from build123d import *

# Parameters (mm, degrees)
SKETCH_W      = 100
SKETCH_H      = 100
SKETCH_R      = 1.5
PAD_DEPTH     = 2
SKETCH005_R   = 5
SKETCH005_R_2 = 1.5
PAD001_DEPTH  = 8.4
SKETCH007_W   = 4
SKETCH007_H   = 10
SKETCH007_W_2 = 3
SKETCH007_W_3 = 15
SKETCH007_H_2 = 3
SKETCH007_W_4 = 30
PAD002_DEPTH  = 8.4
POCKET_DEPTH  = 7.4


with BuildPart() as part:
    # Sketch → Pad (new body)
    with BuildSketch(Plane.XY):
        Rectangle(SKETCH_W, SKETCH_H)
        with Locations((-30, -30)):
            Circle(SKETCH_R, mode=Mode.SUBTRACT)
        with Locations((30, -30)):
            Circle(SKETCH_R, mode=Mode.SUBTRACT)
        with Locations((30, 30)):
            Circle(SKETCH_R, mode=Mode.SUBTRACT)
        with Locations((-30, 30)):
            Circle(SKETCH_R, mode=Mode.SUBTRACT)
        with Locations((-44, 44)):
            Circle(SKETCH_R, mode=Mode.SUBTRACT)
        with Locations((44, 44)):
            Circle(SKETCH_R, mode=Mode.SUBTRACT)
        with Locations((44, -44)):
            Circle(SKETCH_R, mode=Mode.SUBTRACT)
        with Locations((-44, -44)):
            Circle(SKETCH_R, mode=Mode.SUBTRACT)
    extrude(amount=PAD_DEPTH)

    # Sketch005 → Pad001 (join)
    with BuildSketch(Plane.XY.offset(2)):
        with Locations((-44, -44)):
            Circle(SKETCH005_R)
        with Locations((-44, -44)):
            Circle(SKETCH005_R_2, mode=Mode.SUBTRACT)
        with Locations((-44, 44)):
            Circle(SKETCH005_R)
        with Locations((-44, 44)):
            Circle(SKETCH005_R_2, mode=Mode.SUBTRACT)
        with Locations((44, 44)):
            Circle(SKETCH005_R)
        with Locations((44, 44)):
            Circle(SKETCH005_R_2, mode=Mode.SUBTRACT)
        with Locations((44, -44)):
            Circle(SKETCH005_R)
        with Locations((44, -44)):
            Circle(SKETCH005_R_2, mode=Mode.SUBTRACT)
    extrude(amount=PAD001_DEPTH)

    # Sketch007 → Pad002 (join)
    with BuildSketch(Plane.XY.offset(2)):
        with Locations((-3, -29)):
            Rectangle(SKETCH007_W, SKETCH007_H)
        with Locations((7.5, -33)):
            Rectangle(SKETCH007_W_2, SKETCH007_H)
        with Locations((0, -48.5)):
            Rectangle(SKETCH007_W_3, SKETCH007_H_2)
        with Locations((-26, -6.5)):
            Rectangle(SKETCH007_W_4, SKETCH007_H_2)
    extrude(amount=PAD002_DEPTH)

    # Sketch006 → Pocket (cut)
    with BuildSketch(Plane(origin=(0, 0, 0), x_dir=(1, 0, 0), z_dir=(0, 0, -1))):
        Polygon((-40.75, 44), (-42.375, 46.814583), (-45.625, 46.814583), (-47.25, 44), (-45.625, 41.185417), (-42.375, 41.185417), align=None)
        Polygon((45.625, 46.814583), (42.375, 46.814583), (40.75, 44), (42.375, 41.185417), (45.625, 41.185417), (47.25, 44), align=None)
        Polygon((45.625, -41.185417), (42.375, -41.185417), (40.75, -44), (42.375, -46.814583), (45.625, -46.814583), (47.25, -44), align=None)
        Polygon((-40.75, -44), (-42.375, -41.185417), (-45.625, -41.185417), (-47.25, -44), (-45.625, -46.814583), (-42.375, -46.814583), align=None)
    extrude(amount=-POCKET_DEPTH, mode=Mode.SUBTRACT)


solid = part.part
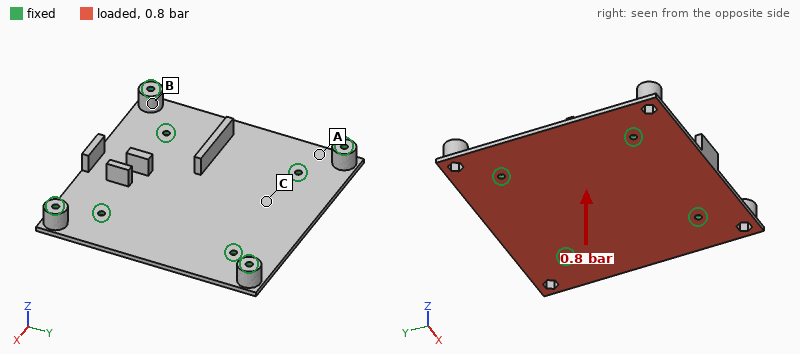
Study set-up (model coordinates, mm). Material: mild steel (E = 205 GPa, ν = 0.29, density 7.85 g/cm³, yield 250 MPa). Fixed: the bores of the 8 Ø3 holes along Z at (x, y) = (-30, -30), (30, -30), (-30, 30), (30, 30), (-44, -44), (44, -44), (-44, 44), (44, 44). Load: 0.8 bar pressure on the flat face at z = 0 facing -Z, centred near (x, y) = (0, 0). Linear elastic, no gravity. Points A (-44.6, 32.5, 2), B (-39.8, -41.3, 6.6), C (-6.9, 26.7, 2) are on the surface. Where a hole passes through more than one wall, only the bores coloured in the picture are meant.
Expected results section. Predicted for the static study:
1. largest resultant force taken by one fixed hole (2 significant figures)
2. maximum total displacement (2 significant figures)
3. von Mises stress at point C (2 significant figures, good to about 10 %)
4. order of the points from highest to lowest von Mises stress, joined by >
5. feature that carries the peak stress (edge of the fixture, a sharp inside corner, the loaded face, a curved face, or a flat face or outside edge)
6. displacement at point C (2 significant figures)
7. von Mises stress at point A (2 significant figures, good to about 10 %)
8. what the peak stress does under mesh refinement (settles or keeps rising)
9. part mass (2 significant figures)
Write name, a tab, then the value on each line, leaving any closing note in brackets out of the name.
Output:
largest resultant force taken by one fixed hole	190 N
maximum total displacement	42 µm
von Mises stress at point C	20 MPa
order of the points from highest to lowest von Mises stress, joined by >	C > A > B
feature that carries the peak stress	edge of the fixture
displacement at point C	27 µm
von Mises stress at point A	12 MPa
what the peak stress does under mesh refinement	keeps rising
part mass	180 g
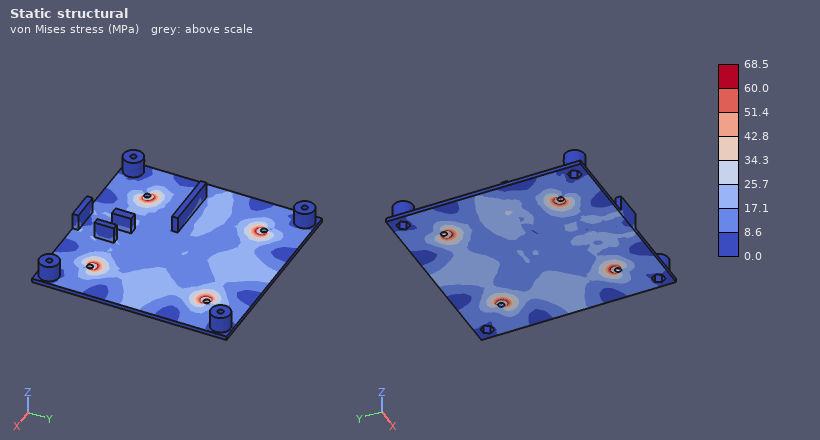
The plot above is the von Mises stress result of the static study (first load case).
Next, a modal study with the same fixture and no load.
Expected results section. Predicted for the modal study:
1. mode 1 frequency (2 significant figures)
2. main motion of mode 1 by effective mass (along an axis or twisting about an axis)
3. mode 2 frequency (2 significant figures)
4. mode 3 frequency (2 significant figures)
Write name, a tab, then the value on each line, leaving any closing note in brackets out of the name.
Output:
mode 1 frequency	2000 Hz
main motion of mode 1 by effective mass	along Z
mode 2 frequency	2100 Hz
mode 3 frequency	2400 Hz
